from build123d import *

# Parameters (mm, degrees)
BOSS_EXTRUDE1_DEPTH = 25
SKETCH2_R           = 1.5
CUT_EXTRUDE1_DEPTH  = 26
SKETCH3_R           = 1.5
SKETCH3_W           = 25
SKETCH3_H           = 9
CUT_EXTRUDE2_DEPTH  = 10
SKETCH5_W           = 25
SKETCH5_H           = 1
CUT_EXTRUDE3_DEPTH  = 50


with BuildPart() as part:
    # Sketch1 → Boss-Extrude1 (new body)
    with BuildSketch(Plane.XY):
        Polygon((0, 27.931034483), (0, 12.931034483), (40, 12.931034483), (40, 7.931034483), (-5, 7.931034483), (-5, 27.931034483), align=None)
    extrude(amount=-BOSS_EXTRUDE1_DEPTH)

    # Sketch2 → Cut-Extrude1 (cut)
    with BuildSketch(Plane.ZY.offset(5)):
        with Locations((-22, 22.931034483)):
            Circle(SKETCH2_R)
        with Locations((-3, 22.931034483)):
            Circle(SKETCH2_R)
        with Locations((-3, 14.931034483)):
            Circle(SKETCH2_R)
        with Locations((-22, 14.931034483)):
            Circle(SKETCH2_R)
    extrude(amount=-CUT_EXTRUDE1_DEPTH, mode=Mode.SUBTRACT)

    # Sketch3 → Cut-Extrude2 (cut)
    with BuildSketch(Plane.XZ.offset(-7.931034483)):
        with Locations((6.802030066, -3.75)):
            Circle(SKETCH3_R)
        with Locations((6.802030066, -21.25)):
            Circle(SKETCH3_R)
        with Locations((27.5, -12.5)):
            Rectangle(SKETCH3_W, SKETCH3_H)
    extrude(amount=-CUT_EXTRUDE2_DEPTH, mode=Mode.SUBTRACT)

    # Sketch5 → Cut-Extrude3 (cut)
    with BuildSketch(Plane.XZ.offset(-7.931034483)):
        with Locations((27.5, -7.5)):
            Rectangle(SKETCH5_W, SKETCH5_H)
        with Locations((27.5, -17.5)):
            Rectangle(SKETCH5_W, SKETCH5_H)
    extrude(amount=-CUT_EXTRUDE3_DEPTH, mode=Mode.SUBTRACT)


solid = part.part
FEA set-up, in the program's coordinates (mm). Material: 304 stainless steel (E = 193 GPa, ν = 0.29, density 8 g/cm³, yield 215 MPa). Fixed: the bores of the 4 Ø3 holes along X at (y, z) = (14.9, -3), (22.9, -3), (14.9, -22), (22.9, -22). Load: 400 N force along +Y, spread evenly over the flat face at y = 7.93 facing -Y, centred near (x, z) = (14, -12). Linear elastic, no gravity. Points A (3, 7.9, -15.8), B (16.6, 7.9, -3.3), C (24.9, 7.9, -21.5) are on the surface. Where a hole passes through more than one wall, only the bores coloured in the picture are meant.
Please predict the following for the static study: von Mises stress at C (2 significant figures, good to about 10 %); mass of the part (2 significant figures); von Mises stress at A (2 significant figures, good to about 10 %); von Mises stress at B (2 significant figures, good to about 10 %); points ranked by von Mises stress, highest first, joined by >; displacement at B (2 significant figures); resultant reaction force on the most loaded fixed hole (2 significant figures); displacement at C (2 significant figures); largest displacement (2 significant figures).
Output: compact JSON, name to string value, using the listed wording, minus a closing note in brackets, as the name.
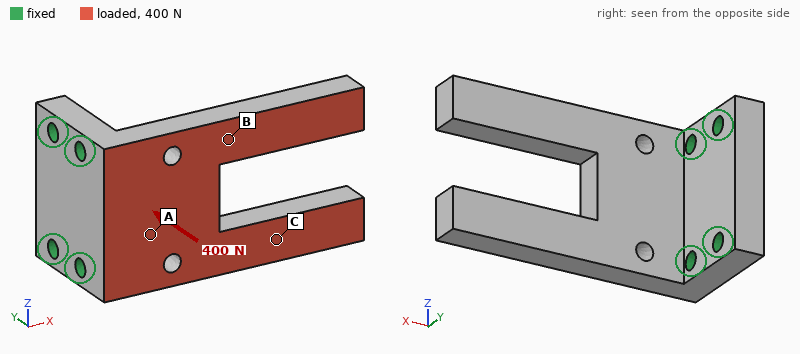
{"von Mises stress at C": "13 MPa", "mass of the part": "47 g", "von Mises stress at A": "46 MPa", "von Mises stress at B": "30 MPa", "points ranked by von Mises stress, highest first, joined by >": "A > B > C", "displacement at B": "28 µm", "resultant reaction force on the most loaded fixed hole": "190 N", "displacement at C": "48 µm", "largest displacement": "88 µm"}
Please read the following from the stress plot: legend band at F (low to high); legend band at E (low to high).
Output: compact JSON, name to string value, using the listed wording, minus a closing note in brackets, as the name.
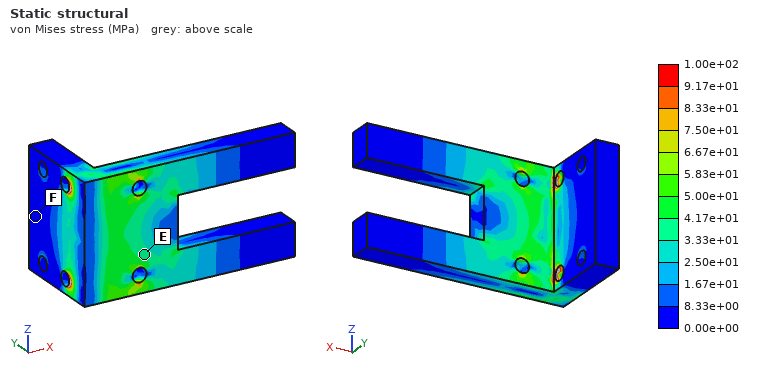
{"legend band at F": "0.00e+00 to 8.33e+00 MPa", "legend band at E": "3.33e+01 to 4.17e+01 MPa"}
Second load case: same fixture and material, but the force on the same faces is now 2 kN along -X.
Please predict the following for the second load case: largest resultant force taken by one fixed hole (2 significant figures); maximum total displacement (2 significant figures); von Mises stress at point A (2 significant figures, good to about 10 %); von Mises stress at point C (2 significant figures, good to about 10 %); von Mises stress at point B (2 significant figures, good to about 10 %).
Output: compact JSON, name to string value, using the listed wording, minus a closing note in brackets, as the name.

{"largest resultant force taken by one fixed hole": "1.2 kN", "maximum total displacement": "100 µm", "von Mises stress at point A": "45 MPa", "von Mises stress at point C": "29 MPa", "von Mises stress at point B": "42 MPa"}
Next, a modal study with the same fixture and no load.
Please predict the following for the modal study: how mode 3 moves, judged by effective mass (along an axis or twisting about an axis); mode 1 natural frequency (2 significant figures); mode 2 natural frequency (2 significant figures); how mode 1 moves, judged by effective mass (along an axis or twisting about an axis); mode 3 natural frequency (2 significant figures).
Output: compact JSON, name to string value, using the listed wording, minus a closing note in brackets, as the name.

{"how mode 3 moves, judged by effective mass": "along Z", "mode 1 natural frequency": "2400 Hz", "mode 2 natural frequency": "3500 Hz", "how mode 1 moves, judged by effective mass": "along Y", "mode 3 natural frequency": "5500 Hz"}
